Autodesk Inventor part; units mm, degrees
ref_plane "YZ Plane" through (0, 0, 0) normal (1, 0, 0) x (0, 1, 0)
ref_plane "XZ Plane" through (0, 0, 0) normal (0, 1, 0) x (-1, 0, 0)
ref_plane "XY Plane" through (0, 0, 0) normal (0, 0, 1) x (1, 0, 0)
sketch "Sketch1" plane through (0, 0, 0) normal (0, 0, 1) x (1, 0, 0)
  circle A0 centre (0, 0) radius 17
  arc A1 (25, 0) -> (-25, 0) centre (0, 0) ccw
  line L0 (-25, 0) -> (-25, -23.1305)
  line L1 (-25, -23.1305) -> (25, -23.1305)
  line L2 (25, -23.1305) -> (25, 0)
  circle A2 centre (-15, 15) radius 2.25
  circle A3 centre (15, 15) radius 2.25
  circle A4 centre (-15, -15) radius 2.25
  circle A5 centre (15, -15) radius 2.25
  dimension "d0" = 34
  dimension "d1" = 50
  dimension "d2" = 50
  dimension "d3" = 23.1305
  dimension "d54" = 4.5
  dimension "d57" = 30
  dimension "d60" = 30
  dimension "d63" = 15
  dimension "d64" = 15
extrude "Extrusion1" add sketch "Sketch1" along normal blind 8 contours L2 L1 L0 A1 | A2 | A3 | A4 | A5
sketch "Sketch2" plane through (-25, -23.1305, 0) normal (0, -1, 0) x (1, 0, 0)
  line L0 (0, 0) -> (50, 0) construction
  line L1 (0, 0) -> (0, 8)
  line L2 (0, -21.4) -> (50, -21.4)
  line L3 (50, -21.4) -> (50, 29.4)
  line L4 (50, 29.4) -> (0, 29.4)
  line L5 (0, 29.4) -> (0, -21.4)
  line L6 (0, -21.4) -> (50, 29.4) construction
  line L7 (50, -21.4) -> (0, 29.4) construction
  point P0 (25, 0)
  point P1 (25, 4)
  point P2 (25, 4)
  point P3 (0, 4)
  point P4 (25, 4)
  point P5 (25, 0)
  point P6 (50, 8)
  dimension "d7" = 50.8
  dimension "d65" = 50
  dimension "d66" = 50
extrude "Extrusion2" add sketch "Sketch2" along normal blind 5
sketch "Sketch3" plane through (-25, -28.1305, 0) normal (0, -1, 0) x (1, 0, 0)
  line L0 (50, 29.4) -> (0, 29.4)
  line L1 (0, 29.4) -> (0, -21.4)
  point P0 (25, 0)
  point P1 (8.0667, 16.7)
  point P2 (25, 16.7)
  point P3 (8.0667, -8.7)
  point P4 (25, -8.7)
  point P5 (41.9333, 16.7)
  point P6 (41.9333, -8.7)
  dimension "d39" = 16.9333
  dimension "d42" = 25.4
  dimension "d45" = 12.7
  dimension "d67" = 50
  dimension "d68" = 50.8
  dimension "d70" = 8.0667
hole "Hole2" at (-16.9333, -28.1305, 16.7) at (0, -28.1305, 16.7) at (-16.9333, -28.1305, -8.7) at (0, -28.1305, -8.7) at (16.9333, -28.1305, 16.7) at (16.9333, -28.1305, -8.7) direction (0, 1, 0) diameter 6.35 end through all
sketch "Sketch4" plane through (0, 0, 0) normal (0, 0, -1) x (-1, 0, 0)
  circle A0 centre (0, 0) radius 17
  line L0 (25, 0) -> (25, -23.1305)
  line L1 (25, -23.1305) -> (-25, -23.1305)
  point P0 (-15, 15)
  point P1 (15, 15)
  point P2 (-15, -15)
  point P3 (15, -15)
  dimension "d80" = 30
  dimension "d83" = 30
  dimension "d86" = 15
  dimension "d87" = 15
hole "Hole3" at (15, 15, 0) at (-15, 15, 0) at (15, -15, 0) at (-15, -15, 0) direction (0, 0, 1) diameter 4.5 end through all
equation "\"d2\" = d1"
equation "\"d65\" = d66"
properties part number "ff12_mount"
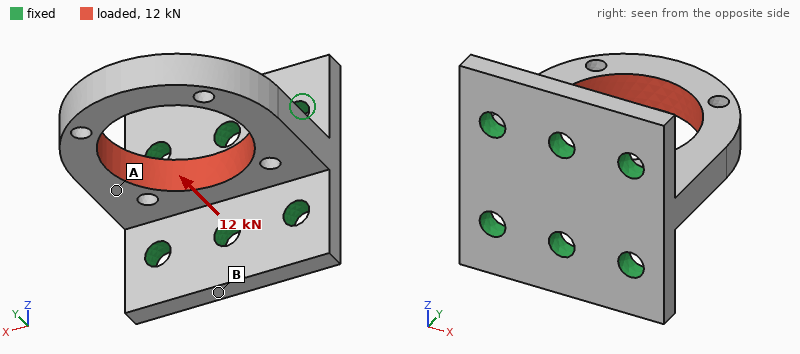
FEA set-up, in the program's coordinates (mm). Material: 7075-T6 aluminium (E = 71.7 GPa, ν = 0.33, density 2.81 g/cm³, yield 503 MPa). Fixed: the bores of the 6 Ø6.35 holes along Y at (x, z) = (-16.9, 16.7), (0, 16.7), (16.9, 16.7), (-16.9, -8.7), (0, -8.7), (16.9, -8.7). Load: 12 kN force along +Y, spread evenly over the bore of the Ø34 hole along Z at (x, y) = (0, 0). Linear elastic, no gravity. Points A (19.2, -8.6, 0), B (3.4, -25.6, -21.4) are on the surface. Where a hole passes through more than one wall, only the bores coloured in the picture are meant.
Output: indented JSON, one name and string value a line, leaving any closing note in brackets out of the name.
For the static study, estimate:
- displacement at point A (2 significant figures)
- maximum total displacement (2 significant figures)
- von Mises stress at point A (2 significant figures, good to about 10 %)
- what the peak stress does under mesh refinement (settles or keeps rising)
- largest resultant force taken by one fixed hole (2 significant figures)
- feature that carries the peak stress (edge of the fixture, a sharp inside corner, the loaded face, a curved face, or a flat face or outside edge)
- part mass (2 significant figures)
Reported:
{
  "displacement at point A": "0.049 mm",
  "maximum total displacement": "0.11 mm",
  "von Mises stress at point A": "75 MPa",
  "what the peak stress does under mesh refinement": "keeps rising",
  "largest resultant force taken by one fixed hole": "2.6 kN",
  "feature that carries the peak stress": "edge of the fixture",
  "part mass": "59 g"
}
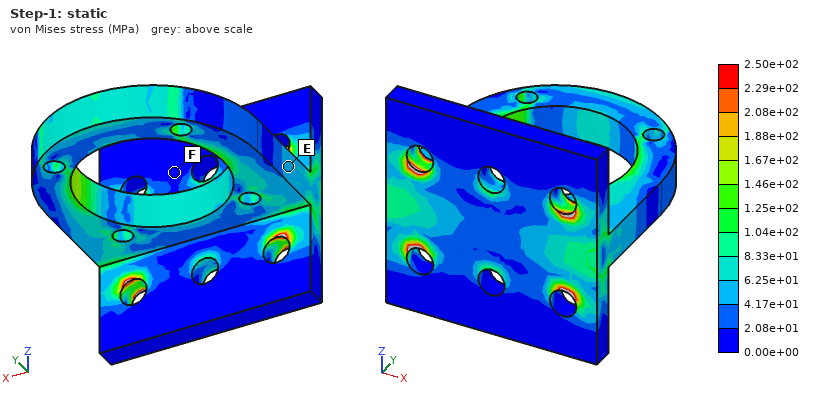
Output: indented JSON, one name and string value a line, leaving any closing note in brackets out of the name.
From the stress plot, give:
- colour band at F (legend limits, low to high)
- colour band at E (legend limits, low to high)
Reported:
{
  "colour band at F": "0.00e+00 to 2.08e+01 MPa",
  "colour band at E": "4.17e+01 to 6.25e+01 MPa"
}
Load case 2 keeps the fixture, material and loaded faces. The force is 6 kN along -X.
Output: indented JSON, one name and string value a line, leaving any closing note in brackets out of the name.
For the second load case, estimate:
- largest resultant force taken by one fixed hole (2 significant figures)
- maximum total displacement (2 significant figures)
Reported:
{
  "largest resultant force taken by one fixed hole": "2.3 kN",
  "maximum total displacement": "0.26 mm"
}
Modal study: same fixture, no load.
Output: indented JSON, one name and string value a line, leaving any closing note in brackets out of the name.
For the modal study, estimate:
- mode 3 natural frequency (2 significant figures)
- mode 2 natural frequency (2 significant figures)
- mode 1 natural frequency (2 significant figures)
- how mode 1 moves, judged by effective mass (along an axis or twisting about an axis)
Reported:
{
  "mode 3 natural frequency": "5900 Hz",
  "mode 2 natural frequency": "5600 Hz",
  "mode 1 natural frequency": "2500 Hz",
  "how mode 1 moves, judged by effective mass": "along Z"
}
